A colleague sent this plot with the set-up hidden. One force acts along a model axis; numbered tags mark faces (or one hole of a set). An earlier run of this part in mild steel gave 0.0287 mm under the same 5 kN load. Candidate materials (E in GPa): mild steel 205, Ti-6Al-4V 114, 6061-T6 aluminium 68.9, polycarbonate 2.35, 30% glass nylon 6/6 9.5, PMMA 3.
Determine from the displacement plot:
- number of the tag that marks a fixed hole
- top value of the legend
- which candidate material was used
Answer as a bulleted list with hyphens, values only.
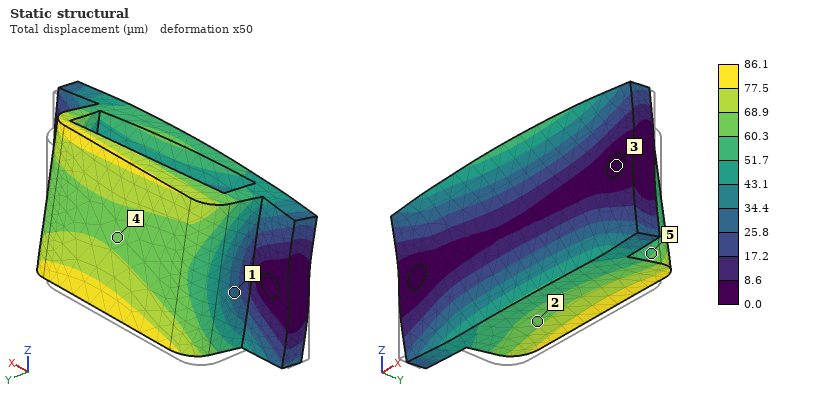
- 3
- 86.1 µm
- 6061-T6 aluminium
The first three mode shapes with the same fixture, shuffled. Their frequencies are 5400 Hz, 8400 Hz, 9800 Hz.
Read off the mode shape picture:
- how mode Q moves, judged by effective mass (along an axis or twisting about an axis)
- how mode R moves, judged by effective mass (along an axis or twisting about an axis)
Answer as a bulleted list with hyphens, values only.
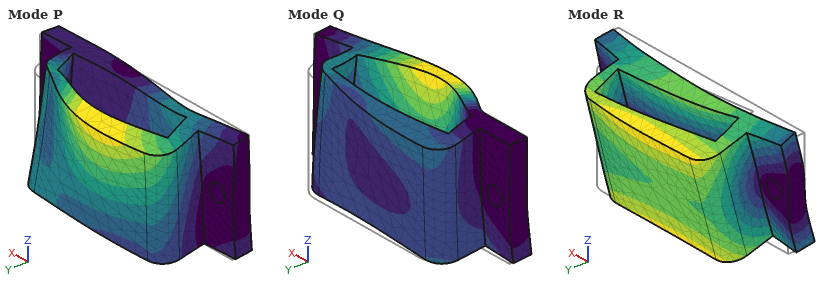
- along Y
- along Z
